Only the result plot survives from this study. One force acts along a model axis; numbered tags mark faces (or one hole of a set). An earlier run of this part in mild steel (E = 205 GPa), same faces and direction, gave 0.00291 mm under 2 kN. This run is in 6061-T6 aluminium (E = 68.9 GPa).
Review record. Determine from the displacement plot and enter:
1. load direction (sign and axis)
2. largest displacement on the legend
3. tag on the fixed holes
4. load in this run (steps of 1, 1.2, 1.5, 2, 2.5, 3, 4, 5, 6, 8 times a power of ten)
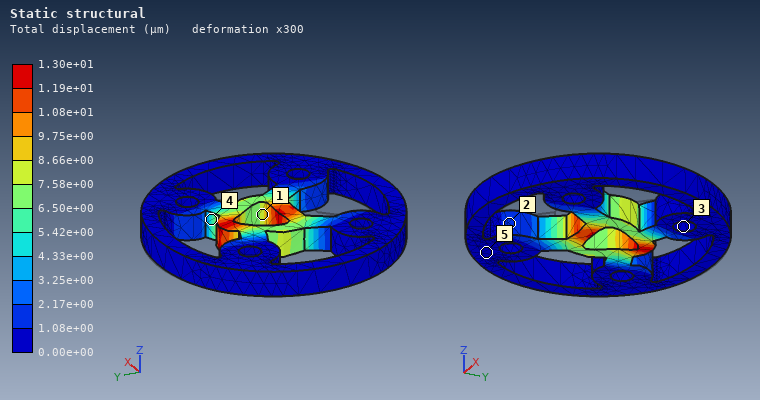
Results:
+Y
1.30e+01 µm
3
3 kN
